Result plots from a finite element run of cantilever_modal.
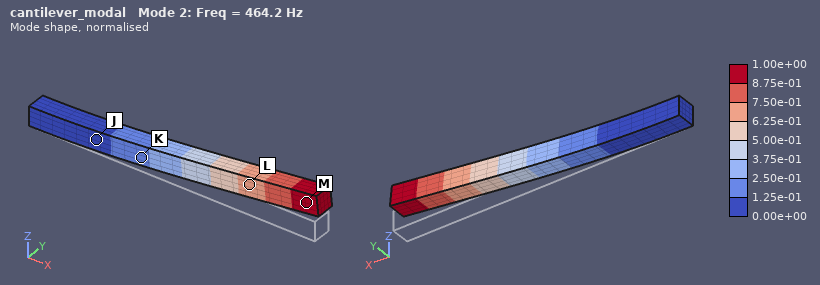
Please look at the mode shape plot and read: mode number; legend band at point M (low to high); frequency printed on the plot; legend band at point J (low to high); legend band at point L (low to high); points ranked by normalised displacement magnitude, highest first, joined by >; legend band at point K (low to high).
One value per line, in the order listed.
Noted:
2
8.75e-01 to 1.00e+00
464.2 Hz
0.00e+00 to 1.25e-01
6.25e-01 to 7.50e-01
M > L > K > J
1.25e-01 to 2.50e-01
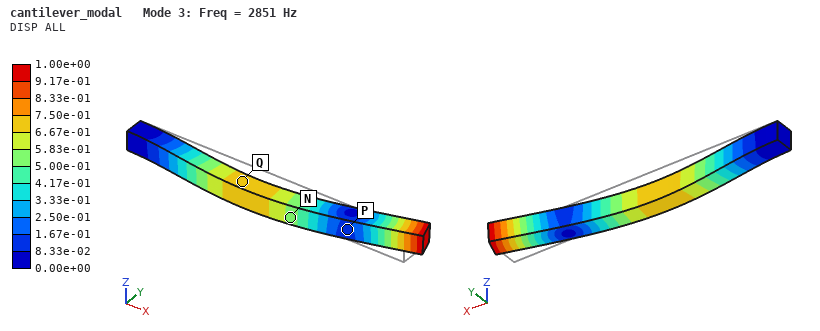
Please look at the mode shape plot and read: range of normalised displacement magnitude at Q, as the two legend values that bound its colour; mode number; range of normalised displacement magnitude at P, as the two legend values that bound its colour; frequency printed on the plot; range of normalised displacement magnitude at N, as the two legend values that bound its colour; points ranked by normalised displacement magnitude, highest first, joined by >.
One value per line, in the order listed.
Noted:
6.67e-01 to 7.50e-01
3
8.33e-02 to 1.67e-01
2851 Hz
5.00e-01 to 5.83e-01
Q > N > P
